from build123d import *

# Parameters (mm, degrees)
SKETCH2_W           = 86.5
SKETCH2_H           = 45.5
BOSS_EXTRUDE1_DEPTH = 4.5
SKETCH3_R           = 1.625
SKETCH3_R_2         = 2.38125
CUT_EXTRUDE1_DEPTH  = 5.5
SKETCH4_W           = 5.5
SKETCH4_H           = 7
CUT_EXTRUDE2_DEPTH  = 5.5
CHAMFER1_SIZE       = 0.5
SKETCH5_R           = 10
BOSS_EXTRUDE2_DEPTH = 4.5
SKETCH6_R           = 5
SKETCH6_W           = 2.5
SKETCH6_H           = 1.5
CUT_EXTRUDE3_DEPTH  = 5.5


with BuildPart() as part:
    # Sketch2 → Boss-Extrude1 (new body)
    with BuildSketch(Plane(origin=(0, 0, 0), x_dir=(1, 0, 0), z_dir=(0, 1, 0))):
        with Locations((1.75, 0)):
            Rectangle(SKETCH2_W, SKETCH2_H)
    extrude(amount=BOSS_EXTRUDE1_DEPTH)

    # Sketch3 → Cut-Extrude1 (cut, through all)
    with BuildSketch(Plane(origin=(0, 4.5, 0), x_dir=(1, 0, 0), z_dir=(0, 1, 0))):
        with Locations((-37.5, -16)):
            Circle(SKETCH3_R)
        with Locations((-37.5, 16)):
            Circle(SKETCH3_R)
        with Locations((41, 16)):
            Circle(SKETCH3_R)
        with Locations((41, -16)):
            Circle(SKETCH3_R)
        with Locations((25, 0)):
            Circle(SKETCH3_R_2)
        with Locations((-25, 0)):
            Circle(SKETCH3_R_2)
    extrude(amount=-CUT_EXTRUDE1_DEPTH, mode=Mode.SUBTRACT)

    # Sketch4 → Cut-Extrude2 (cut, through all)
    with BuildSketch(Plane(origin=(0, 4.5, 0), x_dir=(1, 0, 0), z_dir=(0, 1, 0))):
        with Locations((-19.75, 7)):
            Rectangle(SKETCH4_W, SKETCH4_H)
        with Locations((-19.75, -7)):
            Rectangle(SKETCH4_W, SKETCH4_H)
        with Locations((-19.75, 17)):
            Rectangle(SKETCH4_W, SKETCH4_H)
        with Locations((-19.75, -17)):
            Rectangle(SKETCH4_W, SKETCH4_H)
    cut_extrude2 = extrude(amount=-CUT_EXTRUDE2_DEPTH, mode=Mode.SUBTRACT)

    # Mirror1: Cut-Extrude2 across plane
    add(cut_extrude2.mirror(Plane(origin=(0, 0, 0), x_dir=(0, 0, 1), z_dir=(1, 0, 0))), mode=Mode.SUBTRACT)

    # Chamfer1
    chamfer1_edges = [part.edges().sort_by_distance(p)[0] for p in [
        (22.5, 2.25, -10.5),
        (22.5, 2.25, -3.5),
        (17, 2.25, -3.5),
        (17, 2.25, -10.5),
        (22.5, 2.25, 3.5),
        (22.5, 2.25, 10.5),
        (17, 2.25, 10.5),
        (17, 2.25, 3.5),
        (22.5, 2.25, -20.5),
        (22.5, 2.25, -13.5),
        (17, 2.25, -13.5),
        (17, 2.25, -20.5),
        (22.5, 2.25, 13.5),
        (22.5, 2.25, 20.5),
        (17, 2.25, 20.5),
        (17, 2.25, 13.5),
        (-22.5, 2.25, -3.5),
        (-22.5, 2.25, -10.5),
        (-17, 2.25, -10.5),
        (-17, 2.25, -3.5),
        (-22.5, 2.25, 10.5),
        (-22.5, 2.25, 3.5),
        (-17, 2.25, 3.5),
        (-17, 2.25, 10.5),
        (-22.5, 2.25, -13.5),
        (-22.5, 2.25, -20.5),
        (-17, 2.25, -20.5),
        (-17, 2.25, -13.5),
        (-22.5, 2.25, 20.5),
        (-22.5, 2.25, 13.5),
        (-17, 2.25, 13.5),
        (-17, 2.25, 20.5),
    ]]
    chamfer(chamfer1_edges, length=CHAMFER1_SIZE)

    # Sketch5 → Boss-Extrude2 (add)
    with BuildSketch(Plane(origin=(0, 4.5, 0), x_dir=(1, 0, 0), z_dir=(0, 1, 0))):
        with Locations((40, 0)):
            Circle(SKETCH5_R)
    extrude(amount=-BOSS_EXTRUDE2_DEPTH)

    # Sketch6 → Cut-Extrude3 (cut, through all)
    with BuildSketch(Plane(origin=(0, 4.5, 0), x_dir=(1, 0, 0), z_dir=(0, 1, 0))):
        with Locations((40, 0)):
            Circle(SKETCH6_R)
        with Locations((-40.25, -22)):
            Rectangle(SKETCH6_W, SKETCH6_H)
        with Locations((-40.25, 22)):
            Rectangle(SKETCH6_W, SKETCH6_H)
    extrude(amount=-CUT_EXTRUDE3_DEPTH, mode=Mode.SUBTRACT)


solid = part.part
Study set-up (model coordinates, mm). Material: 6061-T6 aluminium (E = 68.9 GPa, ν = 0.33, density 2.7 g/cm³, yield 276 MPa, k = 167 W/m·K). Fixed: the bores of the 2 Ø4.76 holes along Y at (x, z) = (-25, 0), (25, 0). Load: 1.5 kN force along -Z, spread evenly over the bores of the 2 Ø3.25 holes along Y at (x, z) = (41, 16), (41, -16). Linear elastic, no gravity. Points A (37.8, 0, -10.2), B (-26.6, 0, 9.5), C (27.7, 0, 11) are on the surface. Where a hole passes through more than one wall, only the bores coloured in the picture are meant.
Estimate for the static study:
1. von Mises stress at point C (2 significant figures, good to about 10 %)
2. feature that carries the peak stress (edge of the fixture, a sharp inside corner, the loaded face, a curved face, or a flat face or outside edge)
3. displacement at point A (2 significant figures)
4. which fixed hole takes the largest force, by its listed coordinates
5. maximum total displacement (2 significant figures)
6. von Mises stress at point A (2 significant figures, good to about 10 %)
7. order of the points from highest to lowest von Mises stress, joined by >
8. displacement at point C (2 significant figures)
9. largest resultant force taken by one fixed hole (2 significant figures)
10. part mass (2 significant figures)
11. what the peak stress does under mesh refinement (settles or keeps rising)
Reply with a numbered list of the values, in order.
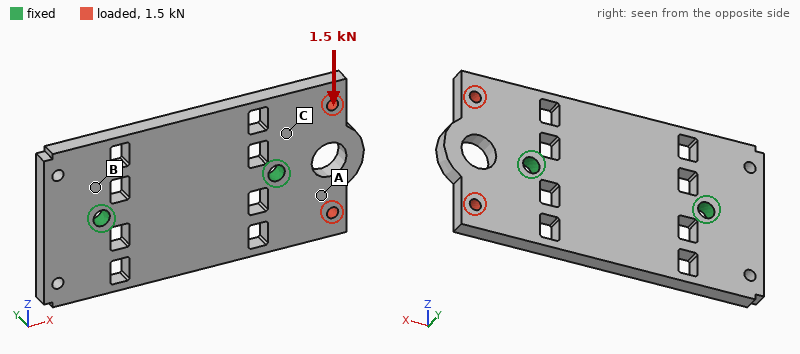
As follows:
1. 11 MPa
2. edge of the fixture
3. 14 µm
4. (25, 0)
5. 26 µm
6. 20 MPa
7. A > C > B
8. 6.3 µm
9. 1.9 kN
10. 43 g
11. keeps rising
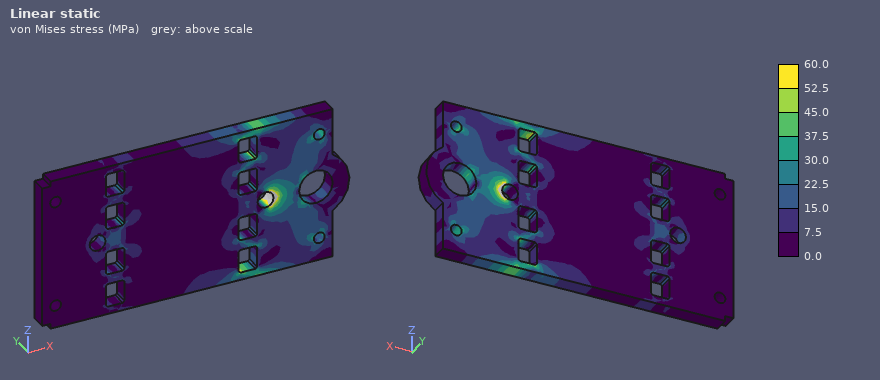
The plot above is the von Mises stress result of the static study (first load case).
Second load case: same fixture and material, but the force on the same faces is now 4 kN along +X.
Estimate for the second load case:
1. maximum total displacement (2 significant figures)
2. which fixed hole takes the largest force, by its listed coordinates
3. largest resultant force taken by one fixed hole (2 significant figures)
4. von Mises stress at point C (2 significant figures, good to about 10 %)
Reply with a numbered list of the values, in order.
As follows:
1. 23 µm
2. (25, 0)
3. 3.0 kN
4. 20 MPa
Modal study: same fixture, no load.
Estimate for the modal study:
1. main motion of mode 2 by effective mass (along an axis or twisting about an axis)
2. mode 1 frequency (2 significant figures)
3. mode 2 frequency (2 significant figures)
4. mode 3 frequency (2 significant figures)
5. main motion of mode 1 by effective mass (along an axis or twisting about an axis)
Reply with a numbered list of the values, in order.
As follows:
1. along Y
2. 4300 Hz
3. 5400 Hz
4. 5700 Hz
5. twisting about X
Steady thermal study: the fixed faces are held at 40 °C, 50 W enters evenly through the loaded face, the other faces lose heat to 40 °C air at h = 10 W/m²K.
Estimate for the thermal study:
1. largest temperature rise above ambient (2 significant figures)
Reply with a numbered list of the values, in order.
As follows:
1. 51 K
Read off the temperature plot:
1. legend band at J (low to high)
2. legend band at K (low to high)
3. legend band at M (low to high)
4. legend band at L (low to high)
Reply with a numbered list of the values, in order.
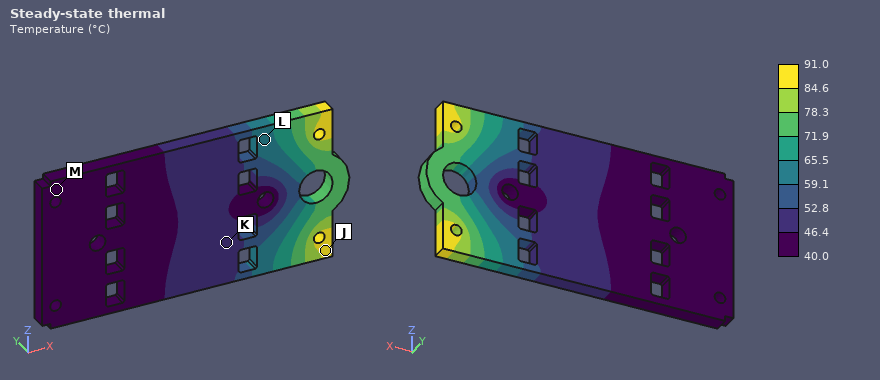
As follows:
1. 84.6 to 91.0 °C
2. 46.4 to 52.8 °C
3. 40.0 to 46.4 °C
4. 59.1 to 65.5 °C
